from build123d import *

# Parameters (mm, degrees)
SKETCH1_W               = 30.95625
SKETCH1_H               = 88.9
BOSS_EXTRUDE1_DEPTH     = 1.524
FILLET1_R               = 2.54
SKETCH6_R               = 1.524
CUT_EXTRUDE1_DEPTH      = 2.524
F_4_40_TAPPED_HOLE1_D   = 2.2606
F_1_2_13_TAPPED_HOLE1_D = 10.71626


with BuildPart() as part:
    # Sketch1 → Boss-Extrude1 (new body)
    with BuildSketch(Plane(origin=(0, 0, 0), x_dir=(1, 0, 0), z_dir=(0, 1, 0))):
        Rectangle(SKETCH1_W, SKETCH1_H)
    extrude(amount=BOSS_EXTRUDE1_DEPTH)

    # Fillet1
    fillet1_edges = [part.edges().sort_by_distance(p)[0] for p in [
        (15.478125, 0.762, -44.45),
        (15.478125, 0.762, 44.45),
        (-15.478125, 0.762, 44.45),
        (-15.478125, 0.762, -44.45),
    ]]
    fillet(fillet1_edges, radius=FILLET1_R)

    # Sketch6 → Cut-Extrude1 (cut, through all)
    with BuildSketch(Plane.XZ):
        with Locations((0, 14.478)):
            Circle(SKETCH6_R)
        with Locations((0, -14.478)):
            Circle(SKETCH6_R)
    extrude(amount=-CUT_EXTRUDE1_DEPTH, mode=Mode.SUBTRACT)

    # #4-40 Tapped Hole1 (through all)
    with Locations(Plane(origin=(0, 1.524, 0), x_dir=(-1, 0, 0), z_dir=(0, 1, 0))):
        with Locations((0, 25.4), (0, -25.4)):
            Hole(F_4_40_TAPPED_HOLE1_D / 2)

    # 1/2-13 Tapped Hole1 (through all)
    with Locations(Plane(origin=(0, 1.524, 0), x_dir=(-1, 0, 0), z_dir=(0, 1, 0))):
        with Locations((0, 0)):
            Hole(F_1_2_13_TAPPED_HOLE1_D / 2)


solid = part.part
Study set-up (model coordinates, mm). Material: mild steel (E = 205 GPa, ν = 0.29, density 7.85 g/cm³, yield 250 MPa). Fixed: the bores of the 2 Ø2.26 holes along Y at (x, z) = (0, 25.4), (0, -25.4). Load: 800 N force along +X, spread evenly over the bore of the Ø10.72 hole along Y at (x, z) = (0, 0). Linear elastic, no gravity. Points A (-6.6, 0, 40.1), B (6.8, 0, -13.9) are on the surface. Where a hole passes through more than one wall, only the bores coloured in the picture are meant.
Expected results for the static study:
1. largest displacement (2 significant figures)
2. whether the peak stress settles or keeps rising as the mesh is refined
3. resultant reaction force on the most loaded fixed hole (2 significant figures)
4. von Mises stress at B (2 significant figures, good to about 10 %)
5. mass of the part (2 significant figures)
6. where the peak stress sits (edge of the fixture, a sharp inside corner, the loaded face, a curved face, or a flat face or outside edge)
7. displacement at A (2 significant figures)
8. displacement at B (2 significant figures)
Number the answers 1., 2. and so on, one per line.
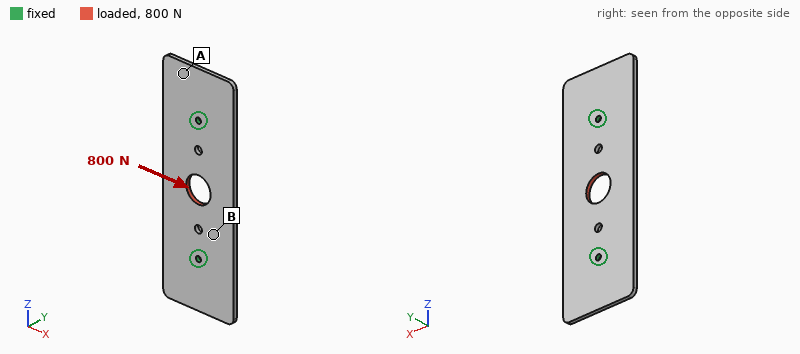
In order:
1. 6.1 µm
2. keeps rising
3. 400 N
4. 22 MPa
5. 32 g
6. edge of the fixture
7. 2.1 µm
8. 3.6 µm
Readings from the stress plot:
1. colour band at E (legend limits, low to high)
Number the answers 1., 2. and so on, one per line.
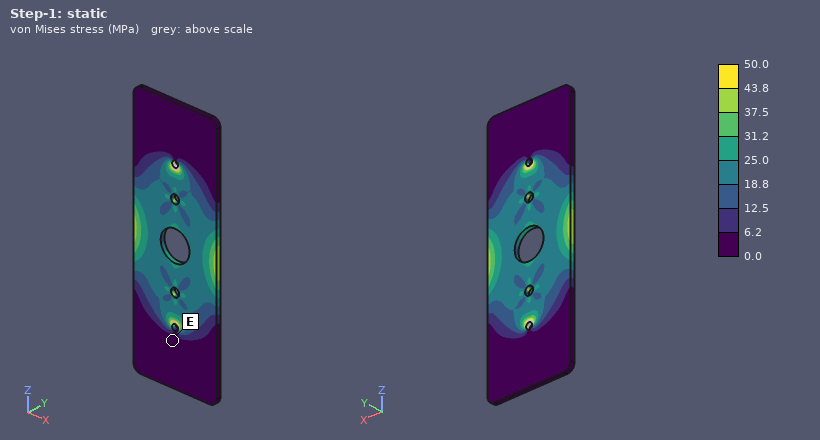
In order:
1. 0.0 to 6.2 MPa
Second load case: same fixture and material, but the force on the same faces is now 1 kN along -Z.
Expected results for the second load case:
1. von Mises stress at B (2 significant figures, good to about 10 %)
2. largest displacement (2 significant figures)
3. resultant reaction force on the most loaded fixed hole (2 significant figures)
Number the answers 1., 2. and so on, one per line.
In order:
1. 13 MPa
2. 2.5 µm
3. 500 N
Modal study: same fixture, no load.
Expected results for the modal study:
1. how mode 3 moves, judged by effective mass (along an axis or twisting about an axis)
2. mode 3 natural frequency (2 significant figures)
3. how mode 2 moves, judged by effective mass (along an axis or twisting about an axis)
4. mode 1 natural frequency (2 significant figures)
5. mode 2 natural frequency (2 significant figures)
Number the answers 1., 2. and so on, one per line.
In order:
1. twisting about X
2. 2900 Hz
3. twisting about Z
4. 2300 Hz
5. 2600 Hz
